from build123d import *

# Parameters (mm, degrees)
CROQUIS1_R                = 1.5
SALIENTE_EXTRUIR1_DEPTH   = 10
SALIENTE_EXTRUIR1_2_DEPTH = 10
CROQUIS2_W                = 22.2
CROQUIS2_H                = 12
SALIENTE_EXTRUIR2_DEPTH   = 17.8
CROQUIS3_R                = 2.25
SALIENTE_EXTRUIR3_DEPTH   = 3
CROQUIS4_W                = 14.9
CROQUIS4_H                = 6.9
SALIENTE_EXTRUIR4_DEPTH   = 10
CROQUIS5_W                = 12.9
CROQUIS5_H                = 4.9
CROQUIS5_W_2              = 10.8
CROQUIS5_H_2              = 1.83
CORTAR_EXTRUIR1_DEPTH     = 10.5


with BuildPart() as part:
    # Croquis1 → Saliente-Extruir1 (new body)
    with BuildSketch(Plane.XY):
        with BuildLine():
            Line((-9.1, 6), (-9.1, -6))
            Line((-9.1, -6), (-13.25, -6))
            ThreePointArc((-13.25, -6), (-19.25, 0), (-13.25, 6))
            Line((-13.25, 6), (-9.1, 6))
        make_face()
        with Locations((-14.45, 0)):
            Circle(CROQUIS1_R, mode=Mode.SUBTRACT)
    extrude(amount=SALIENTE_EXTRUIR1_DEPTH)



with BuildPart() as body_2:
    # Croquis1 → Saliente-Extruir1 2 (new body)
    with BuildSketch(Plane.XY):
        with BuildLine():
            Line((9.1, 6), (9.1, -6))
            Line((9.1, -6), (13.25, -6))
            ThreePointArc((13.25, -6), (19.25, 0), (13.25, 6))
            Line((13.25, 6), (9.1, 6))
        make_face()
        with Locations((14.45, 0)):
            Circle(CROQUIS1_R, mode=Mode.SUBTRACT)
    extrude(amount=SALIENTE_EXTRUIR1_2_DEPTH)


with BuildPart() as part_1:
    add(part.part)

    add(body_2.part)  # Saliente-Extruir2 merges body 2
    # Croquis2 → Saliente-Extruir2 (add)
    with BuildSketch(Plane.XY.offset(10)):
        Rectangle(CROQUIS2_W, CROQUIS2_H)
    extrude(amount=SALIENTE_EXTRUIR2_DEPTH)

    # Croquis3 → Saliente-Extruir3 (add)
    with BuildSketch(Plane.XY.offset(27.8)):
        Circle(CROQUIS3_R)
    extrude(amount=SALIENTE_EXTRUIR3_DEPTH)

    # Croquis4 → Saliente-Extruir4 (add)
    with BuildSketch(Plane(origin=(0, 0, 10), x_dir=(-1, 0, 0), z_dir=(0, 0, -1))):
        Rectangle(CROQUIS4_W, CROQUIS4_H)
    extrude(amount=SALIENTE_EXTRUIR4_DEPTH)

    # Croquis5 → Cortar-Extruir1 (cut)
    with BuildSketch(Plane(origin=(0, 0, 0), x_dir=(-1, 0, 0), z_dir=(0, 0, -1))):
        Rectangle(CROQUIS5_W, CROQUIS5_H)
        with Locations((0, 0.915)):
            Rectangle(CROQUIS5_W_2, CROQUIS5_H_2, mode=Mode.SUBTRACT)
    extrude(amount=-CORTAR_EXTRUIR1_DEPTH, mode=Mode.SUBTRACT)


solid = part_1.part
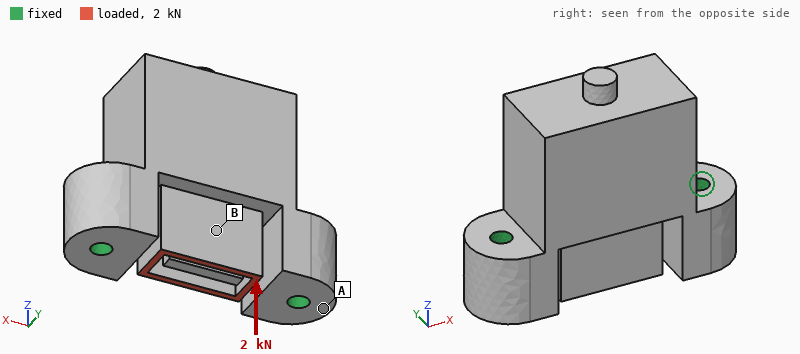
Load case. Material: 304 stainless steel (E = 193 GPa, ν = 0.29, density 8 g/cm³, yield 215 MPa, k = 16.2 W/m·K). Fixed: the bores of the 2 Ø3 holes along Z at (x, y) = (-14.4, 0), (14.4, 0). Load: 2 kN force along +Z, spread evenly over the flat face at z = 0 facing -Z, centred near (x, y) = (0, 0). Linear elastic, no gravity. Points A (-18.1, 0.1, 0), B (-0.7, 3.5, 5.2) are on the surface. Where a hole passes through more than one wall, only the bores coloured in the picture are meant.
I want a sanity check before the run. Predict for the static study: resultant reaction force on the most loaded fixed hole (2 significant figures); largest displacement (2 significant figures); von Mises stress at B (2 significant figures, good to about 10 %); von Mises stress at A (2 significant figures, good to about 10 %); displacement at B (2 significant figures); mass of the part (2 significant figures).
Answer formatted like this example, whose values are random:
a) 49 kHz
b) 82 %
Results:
a) 1.1 kN
b) 5.0 µm
c) 45 MPa
d) 7.6 MPa
e) 3.6 µm
f) 59 g
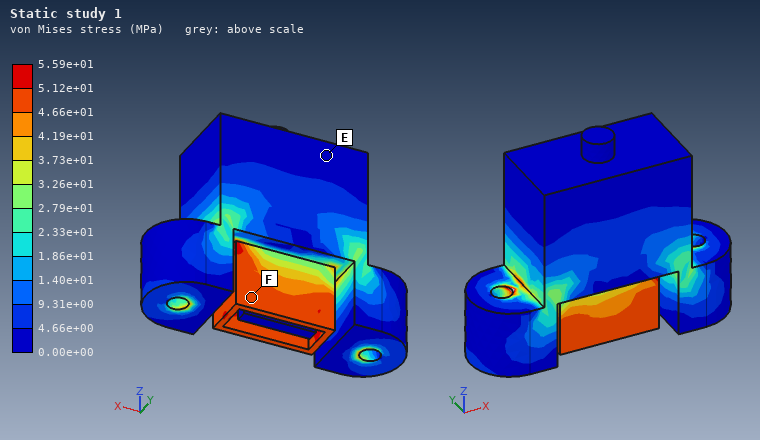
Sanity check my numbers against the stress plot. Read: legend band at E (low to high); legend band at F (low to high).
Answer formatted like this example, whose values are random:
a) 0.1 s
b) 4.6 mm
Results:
a) 0.00e+00 to 4.66e+00 MPa
b) 4.66e+01 to 5.12e+01 MPa
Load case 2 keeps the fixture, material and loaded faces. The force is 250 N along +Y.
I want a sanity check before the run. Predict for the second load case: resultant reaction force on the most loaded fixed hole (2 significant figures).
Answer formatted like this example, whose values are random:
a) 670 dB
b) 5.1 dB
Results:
a) 130 N
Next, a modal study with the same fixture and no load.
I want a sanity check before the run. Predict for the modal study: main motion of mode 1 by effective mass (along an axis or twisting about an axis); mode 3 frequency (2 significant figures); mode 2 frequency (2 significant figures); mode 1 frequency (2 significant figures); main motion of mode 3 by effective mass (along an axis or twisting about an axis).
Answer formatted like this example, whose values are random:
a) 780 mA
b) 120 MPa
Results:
a) along Y
b) 19 kHz
c) 12 kHz
d) 7400 Hz
e) along X
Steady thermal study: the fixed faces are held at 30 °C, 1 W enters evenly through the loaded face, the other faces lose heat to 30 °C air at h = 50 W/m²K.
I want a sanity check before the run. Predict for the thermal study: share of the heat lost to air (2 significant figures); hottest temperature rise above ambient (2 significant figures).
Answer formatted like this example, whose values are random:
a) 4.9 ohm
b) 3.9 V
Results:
a) 60 %
b) 16 K
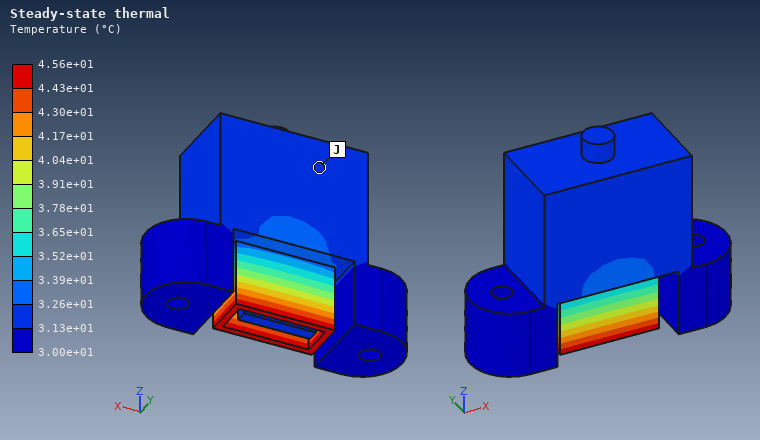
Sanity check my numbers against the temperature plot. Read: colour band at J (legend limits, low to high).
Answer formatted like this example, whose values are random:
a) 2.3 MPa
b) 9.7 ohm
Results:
a) 3.13e+01 to 3.26e+01 °C
